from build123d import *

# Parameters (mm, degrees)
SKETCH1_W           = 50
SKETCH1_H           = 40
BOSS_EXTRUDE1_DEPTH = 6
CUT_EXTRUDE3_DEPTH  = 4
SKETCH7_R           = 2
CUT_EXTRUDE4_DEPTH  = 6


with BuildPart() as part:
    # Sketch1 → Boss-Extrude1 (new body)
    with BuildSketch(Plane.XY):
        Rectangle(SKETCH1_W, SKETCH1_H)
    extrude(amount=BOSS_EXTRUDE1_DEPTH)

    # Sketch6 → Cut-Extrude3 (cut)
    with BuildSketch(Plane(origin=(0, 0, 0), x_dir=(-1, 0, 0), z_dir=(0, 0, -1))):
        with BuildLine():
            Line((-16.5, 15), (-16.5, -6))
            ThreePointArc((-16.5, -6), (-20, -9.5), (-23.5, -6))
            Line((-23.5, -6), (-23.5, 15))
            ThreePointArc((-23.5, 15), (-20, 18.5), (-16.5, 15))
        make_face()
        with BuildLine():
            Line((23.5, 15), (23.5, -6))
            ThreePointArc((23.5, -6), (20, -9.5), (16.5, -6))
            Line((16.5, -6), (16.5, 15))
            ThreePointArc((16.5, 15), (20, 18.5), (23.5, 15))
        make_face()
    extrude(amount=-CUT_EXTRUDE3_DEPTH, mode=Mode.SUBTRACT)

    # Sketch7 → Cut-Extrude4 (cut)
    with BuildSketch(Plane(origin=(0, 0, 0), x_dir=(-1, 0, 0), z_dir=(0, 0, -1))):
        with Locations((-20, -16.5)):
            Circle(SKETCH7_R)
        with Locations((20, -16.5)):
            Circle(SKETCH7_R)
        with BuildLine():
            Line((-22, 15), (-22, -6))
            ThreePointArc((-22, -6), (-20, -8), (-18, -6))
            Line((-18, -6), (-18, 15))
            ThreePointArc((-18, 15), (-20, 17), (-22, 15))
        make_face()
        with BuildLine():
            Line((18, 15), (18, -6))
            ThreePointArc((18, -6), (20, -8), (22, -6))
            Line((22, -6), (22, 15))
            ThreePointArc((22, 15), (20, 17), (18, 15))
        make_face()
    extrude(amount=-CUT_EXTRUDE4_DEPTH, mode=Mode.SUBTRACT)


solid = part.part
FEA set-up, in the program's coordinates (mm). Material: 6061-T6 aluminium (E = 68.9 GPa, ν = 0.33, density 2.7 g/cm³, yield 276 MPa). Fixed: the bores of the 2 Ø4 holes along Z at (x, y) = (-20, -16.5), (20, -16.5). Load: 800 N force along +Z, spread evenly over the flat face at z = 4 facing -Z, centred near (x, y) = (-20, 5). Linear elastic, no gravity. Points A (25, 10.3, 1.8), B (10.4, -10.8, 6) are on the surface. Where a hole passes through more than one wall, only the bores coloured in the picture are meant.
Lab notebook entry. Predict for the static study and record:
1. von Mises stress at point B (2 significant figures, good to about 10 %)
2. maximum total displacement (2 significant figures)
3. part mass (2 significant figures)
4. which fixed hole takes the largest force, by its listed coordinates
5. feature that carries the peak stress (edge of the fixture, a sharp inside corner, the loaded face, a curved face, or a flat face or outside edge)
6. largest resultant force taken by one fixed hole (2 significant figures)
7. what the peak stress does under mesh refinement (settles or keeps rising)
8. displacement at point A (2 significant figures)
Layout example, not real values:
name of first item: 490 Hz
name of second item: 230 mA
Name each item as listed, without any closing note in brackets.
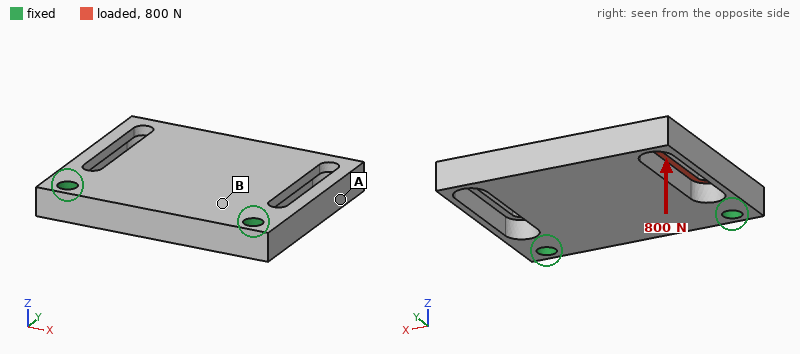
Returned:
von Mises stress at point B: 37 MPa
maximum total displacement: 0.26 mm
part mass: 27 g
which fixed hole takes the largest force, by its listed coordinates: (-20, -16.5)
feature that carries the peak stress: edge of the fixture
largest resultant force taken by one fixed hole: 830 N
what the peak stress does under mesh refinement: keeps rising
displacement at point A: 0.050 mm
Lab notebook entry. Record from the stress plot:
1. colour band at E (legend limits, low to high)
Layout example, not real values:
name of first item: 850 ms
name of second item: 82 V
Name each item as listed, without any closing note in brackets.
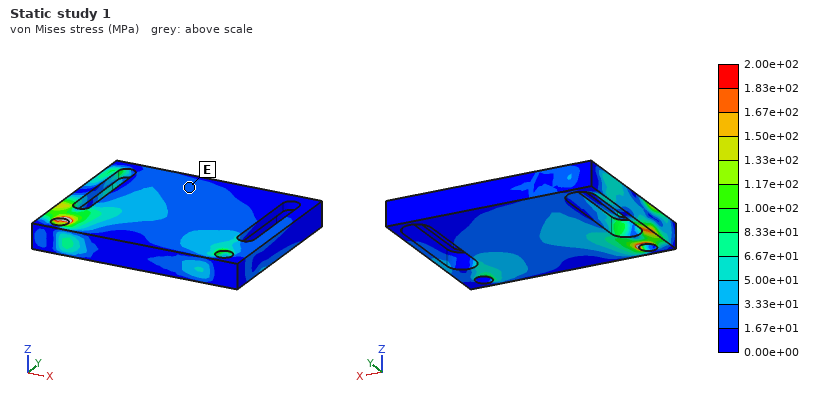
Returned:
colour band at E: 1.67e+01 to 3.33e+01 MPa
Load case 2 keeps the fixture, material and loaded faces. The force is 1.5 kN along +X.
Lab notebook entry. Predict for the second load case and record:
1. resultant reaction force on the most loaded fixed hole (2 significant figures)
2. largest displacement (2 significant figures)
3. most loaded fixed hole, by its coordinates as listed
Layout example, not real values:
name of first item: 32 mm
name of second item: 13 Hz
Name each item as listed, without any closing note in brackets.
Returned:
resultant reaction force on the most loaded fixed hole: 1.2 kN
largest displacement: 0.12 mm
most loaded fixed hole, by its coordinates as listed: (-20, -16.5)
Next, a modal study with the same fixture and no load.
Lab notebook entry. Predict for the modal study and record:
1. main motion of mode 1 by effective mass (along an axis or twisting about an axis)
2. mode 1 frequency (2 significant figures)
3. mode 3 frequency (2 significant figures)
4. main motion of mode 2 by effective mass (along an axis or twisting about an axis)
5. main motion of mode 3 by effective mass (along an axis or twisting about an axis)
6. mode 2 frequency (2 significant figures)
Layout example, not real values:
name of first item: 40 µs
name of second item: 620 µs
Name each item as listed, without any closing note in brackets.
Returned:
main motion of mode 1 by effective mass: along Z
mode 1 frequency: 2900 Hz
mode 3 frequency: 13 kHz
main motion of mode 2 by effective mass: twisting about Y
main motion of mode 3 by effective mass: along X
mode 2 frequency: 7000 Hz
